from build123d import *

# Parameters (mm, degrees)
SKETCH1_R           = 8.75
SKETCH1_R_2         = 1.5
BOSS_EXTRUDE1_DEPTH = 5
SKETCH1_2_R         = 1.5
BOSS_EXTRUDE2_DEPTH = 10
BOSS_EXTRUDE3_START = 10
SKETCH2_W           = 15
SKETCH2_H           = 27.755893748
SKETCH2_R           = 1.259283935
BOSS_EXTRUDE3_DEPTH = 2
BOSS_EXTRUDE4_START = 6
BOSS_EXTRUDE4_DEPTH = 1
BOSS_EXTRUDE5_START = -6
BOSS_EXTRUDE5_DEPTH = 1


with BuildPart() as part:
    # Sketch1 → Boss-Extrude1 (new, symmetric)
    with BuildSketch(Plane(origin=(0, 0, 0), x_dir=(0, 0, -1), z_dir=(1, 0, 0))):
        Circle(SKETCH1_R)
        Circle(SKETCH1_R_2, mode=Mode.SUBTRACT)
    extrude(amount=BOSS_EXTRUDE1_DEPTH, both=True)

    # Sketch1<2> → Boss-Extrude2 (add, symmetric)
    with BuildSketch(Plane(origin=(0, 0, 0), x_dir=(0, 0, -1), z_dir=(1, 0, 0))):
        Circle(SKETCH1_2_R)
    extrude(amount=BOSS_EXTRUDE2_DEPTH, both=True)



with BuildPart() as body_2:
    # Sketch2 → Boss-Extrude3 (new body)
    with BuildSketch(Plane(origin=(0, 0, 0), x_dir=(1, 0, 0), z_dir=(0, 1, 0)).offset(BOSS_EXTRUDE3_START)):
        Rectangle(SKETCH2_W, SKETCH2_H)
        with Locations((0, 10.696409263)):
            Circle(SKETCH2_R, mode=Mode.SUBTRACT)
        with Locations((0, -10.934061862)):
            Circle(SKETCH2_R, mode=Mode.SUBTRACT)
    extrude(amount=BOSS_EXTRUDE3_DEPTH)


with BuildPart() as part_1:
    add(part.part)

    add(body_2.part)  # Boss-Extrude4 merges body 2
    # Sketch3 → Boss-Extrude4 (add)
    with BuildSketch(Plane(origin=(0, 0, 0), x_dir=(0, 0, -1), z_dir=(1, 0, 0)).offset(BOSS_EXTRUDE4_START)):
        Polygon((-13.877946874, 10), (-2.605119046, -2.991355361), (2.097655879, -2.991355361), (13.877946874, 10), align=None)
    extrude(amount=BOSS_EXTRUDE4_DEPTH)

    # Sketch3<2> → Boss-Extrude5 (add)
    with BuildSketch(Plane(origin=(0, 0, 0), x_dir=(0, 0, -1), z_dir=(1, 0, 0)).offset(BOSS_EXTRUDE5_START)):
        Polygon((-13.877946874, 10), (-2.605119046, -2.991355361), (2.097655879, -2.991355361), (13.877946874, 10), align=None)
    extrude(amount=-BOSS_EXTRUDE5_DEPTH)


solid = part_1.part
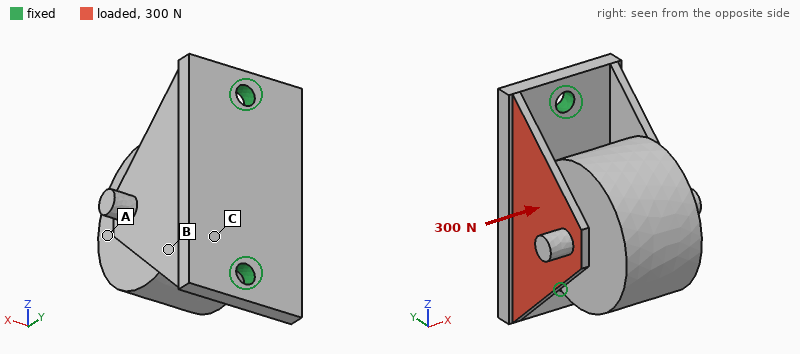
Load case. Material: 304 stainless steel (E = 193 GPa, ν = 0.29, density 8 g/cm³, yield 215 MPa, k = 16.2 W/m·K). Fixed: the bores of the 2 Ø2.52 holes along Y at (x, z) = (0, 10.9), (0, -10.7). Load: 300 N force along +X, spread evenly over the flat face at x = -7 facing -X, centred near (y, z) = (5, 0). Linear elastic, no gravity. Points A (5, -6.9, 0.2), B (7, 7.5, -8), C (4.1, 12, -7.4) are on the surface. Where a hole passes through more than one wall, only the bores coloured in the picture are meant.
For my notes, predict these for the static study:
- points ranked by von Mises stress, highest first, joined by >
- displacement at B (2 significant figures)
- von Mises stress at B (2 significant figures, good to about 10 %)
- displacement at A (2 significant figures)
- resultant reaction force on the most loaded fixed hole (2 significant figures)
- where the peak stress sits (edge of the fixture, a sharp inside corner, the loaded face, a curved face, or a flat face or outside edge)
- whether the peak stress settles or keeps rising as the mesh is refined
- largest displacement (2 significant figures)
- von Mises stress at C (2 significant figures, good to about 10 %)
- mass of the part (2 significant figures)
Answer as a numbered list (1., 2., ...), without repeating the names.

1. B > C > A
2. 9.7 µm
3. 57 MPa
4. 47 µm
5. 150 N
6. edge of the fixture
7. keeps rising
8. 49 µm
9. 26 MPa
10. 30 g
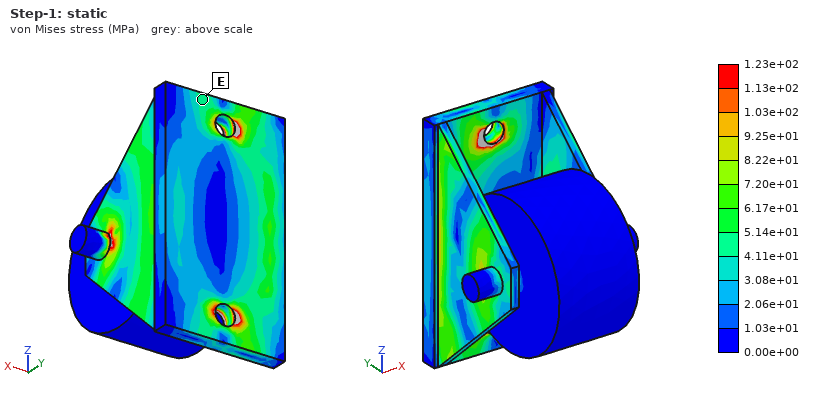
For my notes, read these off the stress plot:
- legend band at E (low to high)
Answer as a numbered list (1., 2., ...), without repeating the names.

1. 4.11e+01 to 5.14e+01 MPa
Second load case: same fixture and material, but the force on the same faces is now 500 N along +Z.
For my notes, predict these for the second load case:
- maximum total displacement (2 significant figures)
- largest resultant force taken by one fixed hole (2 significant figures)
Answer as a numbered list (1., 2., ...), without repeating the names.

1. 12 µm
2. 320 N
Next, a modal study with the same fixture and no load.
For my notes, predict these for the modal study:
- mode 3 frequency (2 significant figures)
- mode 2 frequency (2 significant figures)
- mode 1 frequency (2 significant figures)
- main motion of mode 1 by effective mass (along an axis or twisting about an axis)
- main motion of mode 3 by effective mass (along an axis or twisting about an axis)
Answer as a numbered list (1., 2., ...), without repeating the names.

1. 7400 Hz
2. 4200 Hz
3. 2000 Hz
4. along X
5. along Z
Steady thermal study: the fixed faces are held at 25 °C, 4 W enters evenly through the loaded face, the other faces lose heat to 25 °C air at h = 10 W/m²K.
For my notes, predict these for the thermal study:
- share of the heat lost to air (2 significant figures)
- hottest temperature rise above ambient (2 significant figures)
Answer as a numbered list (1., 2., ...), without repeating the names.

1. 20 %
2. 66 K
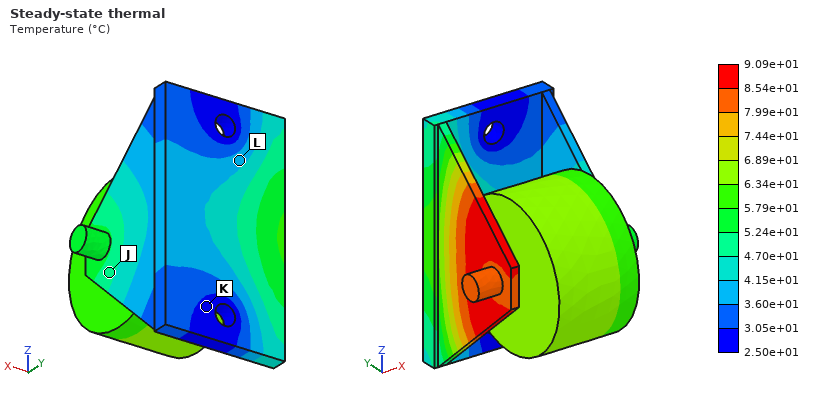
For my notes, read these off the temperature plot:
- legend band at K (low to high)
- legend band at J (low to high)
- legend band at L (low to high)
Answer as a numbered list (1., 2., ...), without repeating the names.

1. 2.50e+01 to 3.05e+01 °C
2. 4.70e+01 to 5.24e+01 °C
3. 3.60e+01 to 4.15e+01 °C
